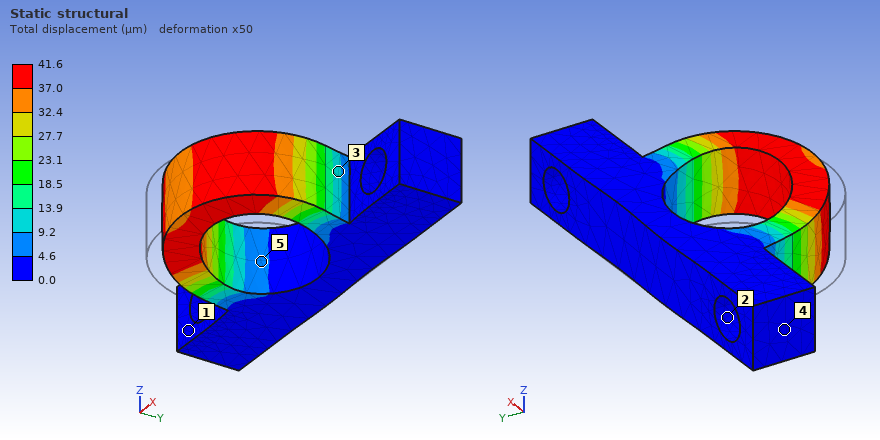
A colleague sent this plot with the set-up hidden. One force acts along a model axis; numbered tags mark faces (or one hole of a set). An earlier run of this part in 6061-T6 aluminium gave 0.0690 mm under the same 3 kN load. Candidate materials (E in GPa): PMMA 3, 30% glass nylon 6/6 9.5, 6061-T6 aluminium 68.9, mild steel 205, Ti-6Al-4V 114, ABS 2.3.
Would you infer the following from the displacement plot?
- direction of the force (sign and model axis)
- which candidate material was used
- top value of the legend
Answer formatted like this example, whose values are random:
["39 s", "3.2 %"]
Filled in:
["+X", "Ti-6Al-4V", "41.6 µm"]
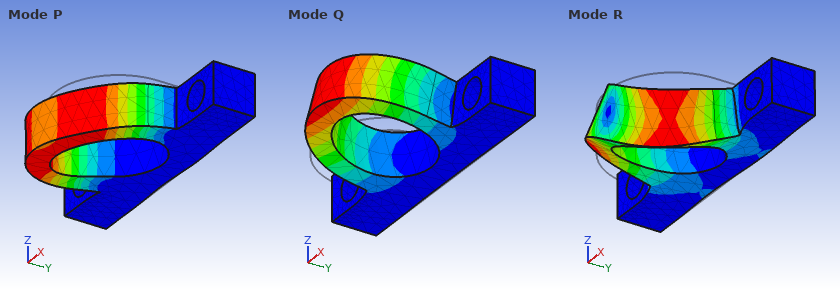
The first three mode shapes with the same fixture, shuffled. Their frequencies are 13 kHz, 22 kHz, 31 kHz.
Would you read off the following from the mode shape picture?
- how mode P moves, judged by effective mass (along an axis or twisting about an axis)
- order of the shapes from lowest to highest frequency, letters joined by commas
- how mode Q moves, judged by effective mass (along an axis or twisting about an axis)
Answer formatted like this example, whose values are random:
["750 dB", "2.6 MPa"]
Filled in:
["along X", "Q, P, R", "along Z"]
